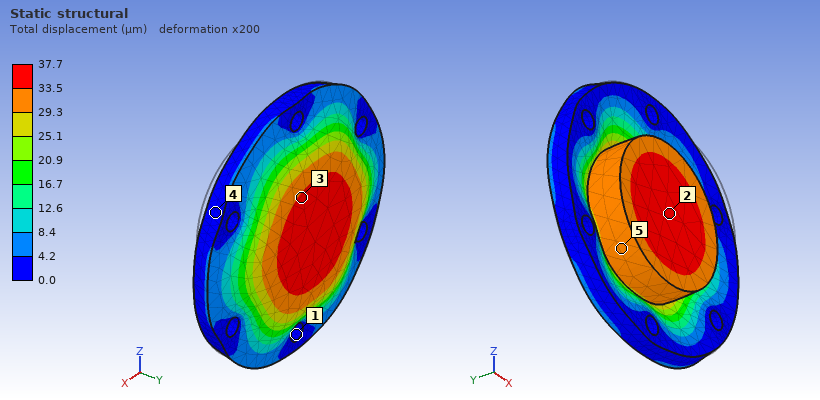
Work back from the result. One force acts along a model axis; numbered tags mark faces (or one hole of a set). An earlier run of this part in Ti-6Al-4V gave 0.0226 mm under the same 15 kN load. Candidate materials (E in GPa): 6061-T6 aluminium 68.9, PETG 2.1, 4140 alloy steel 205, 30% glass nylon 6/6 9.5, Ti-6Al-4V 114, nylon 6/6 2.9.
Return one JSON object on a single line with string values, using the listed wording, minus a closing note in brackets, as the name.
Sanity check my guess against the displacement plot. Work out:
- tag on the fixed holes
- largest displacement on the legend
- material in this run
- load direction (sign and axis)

{"tag on the fixed holes": "1", "largest displacement on the legend": "37.7 µm", "material in this run": "6061-T6 aluminium", "load direction": "+Y"}
